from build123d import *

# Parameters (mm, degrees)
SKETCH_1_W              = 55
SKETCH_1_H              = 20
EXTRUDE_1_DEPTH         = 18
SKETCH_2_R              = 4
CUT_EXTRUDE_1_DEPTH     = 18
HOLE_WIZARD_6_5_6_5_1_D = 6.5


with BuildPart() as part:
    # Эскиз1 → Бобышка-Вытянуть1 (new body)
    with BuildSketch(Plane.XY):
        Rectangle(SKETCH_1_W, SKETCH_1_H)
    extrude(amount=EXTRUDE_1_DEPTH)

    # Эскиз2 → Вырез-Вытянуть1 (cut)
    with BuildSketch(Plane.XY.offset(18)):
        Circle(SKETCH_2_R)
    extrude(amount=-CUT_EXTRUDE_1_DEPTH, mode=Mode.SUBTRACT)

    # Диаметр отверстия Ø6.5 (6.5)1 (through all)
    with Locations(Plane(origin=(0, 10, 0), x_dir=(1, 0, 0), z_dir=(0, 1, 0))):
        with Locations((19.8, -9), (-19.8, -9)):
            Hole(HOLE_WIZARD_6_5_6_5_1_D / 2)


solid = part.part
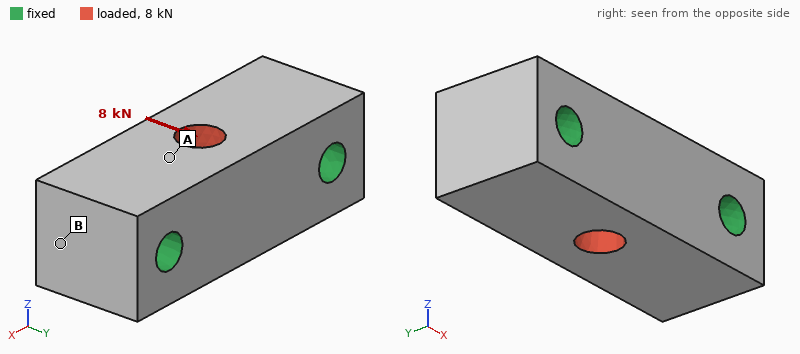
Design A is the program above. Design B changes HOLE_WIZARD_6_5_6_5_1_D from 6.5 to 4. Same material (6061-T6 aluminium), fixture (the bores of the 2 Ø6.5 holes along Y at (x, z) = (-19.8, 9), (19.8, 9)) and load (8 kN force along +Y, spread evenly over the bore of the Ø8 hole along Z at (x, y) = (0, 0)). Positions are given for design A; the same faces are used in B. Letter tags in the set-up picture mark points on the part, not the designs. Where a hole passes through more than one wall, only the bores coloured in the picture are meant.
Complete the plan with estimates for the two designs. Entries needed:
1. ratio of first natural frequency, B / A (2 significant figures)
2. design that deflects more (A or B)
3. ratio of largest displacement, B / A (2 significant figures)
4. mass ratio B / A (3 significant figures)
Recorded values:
0.80
B
1.2
1.05
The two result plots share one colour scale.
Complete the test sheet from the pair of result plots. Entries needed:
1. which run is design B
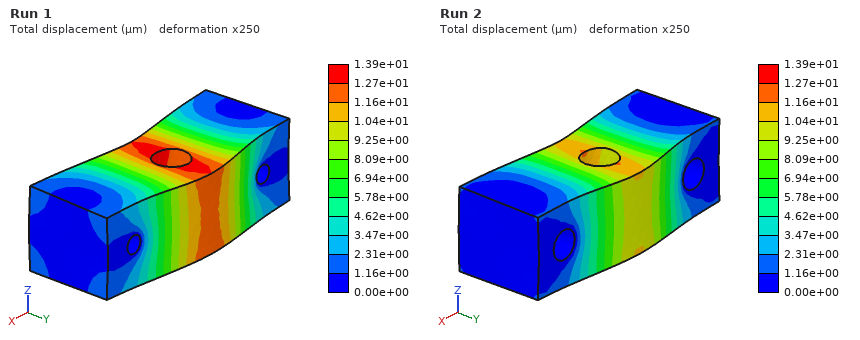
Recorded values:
Run 1
